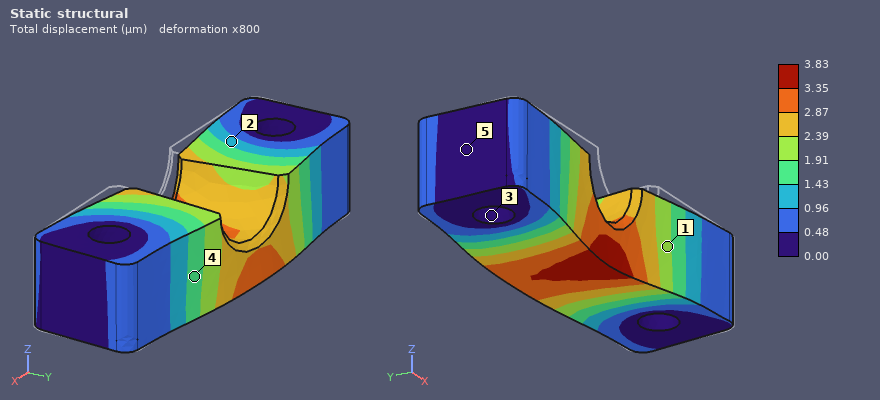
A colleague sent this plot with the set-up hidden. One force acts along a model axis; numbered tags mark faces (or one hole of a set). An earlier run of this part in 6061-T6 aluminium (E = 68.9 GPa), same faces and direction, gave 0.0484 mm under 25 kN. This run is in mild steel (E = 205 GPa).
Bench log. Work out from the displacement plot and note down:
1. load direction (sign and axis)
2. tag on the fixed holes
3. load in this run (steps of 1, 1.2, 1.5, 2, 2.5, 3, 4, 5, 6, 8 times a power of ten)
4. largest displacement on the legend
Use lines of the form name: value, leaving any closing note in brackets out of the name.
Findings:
load direction: +Y
tag on the fixed holes: 3
load in this run: 6 kN
largest displacement on the legend: 3.83 µm
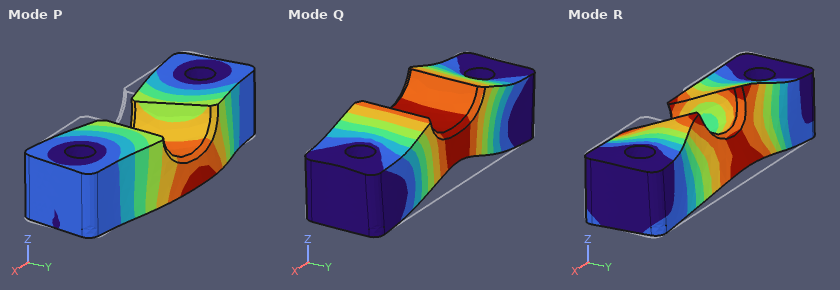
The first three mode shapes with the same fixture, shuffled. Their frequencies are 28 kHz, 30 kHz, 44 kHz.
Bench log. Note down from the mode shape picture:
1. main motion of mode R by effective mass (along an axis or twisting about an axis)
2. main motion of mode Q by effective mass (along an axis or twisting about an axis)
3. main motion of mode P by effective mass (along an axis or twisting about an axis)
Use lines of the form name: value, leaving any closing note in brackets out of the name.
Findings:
main motion of mode R by effective mass: twisting about X
main motion of mode Q by effective mass: along Z
main motion of mode P by effective mass: along Y
